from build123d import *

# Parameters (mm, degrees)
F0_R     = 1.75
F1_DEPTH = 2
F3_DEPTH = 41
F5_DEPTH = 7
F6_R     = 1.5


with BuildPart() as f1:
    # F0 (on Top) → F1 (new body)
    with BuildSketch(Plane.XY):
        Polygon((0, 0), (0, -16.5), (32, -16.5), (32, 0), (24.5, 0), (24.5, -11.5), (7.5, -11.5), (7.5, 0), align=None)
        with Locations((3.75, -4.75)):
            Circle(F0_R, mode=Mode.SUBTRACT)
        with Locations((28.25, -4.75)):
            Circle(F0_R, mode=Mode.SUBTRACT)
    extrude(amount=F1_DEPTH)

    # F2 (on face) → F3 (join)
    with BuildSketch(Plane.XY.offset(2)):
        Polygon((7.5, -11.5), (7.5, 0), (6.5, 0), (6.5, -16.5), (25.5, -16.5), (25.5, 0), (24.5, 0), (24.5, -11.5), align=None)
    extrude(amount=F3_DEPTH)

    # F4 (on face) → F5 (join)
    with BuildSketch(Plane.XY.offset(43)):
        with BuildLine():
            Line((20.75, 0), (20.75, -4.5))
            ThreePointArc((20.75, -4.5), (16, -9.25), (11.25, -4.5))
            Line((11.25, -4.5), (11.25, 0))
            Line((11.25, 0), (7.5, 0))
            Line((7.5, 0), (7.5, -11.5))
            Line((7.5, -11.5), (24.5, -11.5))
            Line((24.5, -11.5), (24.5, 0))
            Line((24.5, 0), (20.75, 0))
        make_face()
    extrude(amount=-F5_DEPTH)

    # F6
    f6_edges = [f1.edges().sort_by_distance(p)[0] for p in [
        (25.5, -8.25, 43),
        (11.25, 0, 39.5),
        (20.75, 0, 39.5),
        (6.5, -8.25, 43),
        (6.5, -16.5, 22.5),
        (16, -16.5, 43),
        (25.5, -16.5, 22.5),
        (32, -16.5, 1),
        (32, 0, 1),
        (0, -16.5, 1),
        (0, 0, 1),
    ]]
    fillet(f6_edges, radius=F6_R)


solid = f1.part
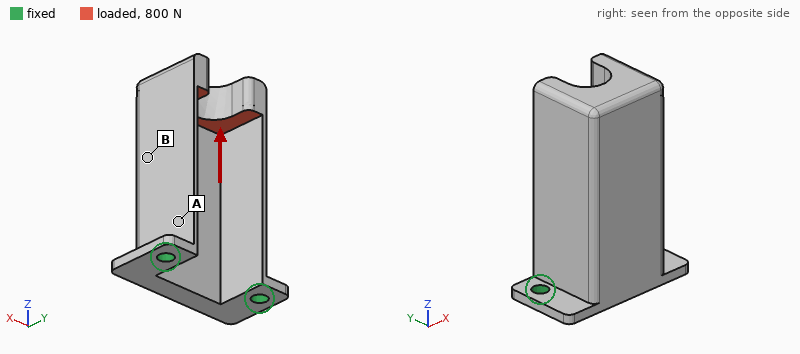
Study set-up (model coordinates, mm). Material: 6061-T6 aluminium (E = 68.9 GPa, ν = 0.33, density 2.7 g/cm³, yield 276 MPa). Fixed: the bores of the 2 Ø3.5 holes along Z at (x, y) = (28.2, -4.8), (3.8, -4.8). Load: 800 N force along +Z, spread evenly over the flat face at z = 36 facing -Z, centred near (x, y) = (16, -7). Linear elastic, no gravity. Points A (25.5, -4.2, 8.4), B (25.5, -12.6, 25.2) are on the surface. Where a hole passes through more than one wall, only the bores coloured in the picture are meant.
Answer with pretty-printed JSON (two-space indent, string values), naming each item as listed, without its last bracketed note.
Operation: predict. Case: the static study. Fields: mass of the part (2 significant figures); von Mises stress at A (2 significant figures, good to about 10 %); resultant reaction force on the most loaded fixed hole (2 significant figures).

{
  "mass of the part": "17 g",
  "von Mises stress at A": "35 MPa",
  "resultant reaction force on the most loaded fixed hole": "400 N"
}
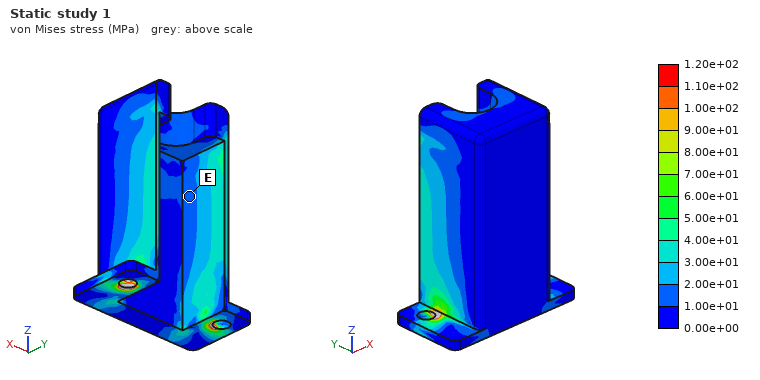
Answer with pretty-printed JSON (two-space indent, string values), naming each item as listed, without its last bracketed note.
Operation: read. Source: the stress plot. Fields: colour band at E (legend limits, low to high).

{
  "colour band at E": "1.00e+01 to 2.00e+01 MPa"
}
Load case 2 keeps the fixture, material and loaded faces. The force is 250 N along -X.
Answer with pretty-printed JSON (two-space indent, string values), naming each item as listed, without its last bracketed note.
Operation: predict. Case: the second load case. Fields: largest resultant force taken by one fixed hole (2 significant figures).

{
  "largest resultant force taken by one fixed hole": "450 N"
}
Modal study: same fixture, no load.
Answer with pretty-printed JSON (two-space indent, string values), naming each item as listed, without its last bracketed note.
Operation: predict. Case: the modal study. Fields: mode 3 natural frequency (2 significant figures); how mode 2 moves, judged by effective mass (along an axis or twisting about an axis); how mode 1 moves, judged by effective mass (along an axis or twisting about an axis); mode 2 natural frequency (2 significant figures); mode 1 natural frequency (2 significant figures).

{
  "mode 3 natural frequency": "7300 Hz",
  "how mode 2 moves, judged by effective mass": "along X",
  "how mode 1 moves, judged by effective mass": "along Y",
  "mode 2 natural frequency": "2600 Hz",
  "mode 1 natural frequency": "1200 Hz"
}
